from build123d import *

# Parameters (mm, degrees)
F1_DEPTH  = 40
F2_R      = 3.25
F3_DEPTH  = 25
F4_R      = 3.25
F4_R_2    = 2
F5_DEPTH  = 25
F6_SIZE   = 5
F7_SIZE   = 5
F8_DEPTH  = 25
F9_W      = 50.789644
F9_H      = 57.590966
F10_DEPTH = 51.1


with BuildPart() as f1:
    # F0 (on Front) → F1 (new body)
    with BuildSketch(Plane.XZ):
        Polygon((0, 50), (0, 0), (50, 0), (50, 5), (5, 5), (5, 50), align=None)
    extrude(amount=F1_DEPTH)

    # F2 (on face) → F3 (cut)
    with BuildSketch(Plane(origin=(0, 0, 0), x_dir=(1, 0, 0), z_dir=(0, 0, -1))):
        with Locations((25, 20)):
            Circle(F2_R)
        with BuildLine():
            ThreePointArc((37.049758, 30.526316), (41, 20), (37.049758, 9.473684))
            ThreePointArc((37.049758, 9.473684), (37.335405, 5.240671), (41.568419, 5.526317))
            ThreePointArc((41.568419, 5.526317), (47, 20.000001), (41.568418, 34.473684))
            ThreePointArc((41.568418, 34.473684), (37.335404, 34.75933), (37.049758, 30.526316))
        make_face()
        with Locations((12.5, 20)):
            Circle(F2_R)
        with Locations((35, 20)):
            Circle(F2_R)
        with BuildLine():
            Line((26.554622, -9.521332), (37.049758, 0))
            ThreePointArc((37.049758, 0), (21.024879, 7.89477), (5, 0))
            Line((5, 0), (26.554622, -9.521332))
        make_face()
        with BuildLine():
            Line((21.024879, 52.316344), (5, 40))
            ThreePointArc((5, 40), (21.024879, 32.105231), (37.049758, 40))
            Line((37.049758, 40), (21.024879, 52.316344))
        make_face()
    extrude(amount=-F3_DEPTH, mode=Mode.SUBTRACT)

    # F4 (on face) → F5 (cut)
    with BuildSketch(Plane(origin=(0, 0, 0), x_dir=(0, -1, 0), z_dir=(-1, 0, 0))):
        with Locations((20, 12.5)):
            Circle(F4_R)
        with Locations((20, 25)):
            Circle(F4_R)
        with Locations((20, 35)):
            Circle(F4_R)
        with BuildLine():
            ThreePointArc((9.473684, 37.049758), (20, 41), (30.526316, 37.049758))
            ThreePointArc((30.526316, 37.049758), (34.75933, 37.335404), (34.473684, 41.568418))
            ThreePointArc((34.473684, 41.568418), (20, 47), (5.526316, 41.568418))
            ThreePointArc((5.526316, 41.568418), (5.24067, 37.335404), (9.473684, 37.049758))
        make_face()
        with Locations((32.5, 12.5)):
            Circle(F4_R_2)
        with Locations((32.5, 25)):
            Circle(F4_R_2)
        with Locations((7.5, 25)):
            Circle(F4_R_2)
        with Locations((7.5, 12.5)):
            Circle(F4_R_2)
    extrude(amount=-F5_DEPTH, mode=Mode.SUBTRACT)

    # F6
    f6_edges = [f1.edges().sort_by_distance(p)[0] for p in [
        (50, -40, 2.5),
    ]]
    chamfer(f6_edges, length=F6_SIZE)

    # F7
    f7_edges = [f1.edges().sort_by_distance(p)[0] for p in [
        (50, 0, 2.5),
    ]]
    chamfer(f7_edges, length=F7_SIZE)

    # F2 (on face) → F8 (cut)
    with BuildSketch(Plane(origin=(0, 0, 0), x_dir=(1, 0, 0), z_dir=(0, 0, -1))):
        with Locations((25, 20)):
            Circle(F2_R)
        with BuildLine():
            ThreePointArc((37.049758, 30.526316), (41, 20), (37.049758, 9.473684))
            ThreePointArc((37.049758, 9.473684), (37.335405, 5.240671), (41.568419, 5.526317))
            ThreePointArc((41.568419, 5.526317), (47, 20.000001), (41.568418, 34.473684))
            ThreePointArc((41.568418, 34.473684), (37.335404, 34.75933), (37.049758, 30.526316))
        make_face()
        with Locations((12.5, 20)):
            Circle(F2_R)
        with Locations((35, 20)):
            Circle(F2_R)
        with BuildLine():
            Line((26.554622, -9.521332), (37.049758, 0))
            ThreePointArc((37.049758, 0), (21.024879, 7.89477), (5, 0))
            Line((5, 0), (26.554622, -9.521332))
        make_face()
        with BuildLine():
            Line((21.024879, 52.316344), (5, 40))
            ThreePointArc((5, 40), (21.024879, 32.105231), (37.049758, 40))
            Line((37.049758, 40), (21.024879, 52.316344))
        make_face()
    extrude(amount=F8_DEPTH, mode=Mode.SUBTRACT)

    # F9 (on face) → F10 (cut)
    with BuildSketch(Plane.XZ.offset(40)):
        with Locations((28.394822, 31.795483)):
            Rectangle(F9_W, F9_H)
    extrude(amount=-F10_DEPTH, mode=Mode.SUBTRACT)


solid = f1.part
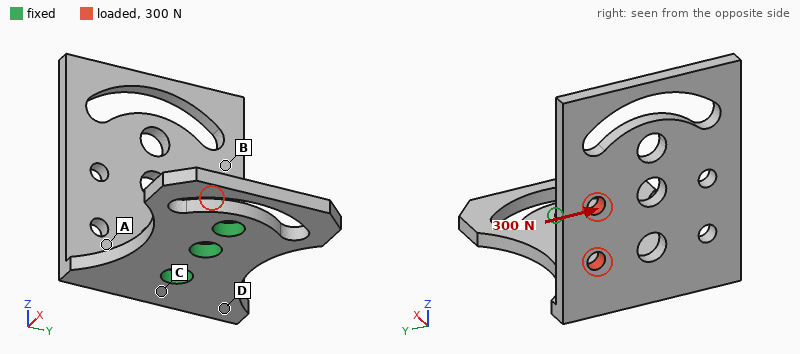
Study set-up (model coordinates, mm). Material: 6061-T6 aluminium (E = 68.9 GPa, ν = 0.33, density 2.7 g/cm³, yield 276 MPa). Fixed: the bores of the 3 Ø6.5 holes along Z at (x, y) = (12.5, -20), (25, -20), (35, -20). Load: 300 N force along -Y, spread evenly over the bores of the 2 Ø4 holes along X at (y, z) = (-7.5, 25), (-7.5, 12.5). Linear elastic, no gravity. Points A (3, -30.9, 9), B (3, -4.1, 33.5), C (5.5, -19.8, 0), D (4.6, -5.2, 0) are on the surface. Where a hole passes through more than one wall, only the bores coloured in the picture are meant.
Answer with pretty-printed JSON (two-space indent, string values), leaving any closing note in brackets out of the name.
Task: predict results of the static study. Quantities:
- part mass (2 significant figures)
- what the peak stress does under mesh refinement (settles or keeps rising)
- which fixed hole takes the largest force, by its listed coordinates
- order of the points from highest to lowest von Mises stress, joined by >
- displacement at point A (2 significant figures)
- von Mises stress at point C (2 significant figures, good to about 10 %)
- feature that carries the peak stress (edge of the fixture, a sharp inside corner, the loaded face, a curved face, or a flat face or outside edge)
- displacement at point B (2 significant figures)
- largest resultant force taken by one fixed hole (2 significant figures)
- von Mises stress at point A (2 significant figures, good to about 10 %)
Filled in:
{
  "part mass": "23 g",
  "what the peak stress does under mesh refinement": "keeps rising",
  "which fixed hole takes the largest force, by its listed coordinates": "(12.5, -20)",
  "order of the points from highest to lowest von Mises stress, joined by >": "C > A > D > B",
  "displacement at point A": "0.067 mm",
  "von Mises stress at point C": "60 MPa",
  "feature that carries the peak stress": "edge of the fixture",
  "displacement at point B": "0.19 mm",
  "largest resultant force taken by one fixed hole": "400 N",
  "von Mises stress at point A": "28 MPa"
}
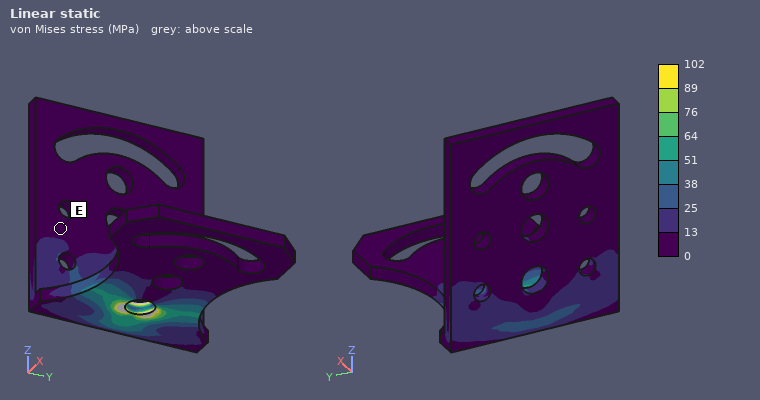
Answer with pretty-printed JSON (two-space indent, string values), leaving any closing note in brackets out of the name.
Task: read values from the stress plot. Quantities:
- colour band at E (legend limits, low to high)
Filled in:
{
  "colour band at E": "0 to 13 MPa"
}
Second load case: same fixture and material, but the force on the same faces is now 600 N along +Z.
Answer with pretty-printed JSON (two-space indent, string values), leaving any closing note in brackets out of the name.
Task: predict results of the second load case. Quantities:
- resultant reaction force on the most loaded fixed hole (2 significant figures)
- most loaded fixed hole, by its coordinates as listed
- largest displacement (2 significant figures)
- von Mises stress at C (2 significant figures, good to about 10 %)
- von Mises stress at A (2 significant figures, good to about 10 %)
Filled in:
{
  "resultant reaction force on the most loaded fixed hole": "690 N",
  "most loaded fixed hole, by its coordinates as listed": "(12.5, -20)",
  "largest displacement": "0.53 mm",
  "von Mises stress at C": "130 MPa",
  "von Mises stress at A": "40 MPa"
}
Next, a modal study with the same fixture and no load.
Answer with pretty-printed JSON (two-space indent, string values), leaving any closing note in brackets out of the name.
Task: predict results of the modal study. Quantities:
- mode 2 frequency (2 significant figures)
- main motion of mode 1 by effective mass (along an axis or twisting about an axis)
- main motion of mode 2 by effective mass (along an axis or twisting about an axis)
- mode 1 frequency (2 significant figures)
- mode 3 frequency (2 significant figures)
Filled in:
{
  "mode 2 frequency": "1500 Hz",
  "main motion of mode 1 by effective mass": "along X",
  "main motion of mode 2 by effective mass": "along Y",
  "mode 1 frequency": "850 Hz",
  "mode 3 frequency": "2600 Hz"
}
